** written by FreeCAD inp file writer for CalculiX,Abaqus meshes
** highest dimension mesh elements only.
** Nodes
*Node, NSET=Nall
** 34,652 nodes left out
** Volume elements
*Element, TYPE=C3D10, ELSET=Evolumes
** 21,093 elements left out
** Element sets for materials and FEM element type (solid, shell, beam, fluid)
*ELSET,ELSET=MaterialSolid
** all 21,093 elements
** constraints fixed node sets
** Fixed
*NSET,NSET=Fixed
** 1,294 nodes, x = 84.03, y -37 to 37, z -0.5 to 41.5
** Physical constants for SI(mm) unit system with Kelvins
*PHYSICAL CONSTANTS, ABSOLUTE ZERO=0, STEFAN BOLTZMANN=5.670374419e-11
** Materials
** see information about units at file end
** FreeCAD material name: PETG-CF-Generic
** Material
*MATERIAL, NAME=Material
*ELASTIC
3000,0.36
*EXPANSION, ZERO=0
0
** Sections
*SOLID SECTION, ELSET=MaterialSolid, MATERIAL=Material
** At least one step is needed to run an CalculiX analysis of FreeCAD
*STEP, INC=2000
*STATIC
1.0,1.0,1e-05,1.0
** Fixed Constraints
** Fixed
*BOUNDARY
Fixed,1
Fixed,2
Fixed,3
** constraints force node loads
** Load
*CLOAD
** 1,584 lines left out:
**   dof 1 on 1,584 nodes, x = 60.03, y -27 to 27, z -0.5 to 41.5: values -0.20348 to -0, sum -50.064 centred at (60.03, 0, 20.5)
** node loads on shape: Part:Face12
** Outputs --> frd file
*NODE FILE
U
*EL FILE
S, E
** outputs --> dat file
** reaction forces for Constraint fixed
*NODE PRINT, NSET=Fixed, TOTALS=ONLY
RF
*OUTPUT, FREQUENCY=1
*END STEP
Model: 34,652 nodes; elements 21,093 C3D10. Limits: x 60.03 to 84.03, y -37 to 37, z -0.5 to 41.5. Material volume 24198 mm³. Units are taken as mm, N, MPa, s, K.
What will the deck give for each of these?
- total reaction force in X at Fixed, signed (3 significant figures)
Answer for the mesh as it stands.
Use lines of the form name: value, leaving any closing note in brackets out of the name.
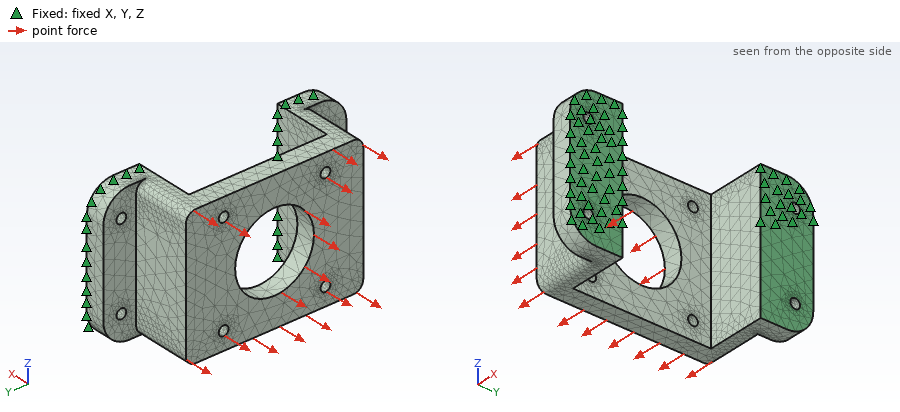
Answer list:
total reaction force in X at Fixed, signed: 50.1 N
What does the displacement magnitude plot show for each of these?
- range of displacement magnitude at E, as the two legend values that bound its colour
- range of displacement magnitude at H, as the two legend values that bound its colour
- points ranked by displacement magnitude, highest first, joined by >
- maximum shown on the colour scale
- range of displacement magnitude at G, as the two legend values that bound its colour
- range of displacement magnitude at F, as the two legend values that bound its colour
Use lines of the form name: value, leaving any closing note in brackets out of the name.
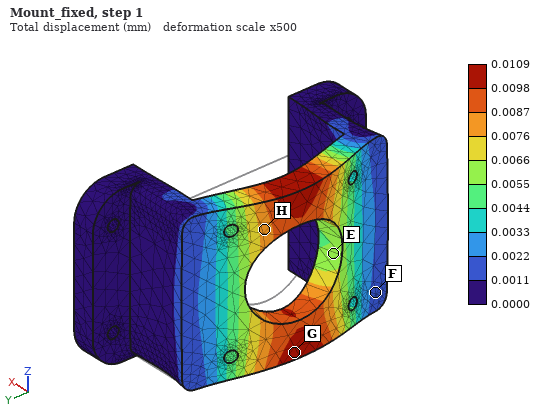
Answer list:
range of displacement magnitude at E, as the two legend values that bound its colour: 0.0055 to 0.0066 mm
range of displacement magnitude at H, as the two legend values that bound its colour: 0.0076 to 0.0087 mm
points ranked by displacement magnitude, highest first, joined by >: G > H > E > F
maximum shown on the colour scale: 0.0109 mm
range of displacement magnitude at G, as the two legend values that bound its colour: 0.0098 to 0.0109 mm
range of displacement magnitude at F, as the two legend values that bound its colour: 0.0011 to 0.0022 mm
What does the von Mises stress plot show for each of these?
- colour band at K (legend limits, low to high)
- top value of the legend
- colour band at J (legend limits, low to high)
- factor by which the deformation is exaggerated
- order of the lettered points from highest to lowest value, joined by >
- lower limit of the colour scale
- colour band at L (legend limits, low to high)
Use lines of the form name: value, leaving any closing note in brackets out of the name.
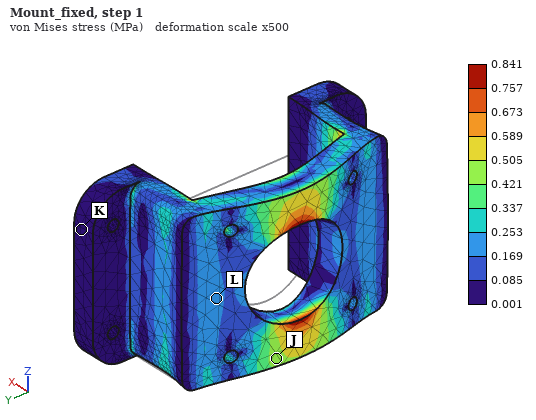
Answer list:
colour band at K: 0.001 to 0.085 MPa
top value of the legend: 0.841 MPa
colour band at J: 0.421 to 0.505 MPa
factor by which the deformation is exaggerated: 500
order of the lettered points from highest to lowest value, joined by >: J > L > K
lower limit of the colour scale: 0.001 MPa
colour band at L: 0.169 to 0.253 MPa
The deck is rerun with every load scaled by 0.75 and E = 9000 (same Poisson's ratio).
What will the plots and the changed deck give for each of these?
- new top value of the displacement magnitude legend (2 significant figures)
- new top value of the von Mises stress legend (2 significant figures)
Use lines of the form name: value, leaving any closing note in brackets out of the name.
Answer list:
new top value of the displacement magnitude legend: 0.0027 mm
new top value of the von Mises stress legend: 0.63 MPa
